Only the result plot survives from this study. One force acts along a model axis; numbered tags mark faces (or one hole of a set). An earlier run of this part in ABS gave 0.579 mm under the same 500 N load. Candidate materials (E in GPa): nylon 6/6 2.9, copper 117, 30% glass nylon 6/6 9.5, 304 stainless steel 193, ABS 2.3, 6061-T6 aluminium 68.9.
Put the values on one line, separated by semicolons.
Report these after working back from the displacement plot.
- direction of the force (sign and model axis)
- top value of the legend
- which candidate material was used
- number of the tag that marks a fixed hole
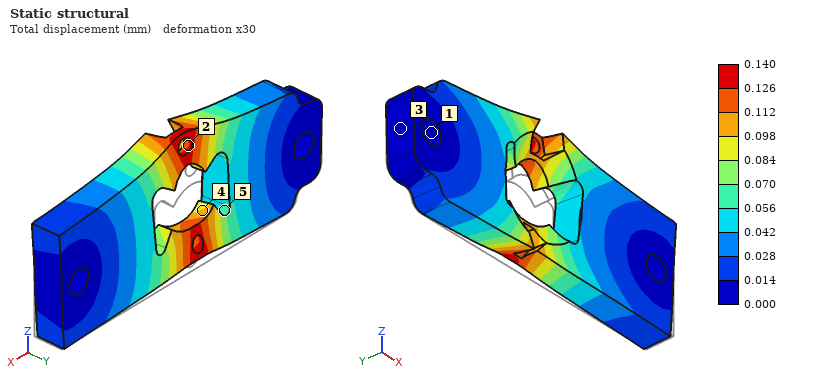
+Z; 0.140 mm; 30% glass nylon 6/6; 1
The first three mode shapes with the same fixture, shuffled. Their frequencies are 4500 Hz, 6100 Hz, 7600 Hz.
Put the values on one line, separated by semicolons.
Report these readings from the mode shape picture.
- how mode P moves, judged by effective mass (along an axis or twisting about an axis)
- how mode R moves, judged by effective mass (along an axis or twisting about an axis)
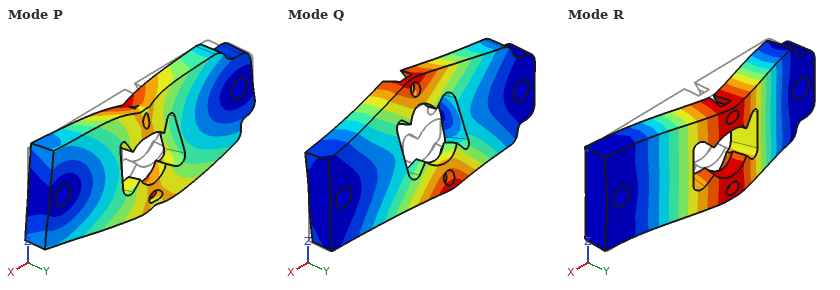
along Z; along Y
